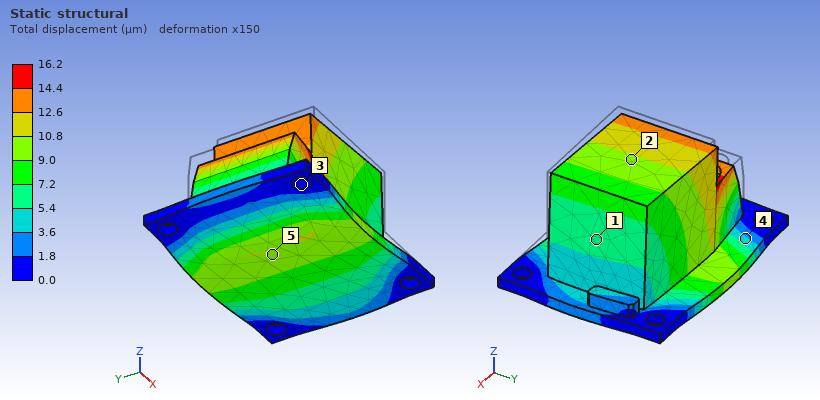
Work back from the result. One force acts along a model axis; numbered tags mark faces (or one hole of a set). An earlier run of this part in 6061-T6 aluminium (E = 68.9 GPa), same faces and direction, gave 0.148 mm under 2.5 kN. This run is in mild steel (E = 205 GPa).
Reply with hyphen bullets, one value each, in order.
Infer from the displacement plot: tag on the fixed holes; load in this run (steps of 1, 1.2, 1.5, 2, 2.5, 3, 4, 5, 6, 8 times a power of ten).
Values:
- 3
- 800 N
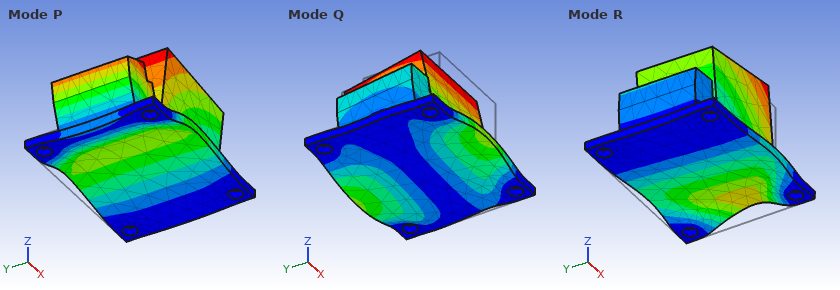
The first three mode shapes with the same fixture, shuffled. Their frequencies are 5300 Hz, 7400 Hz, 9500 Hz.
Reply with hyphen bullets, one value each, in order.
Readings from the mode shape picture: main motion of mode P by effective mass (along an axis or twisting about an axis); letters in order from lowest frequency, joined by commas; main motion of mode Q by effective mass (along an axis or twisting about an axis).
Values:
- along Z
- P, Q, R
- along Y
